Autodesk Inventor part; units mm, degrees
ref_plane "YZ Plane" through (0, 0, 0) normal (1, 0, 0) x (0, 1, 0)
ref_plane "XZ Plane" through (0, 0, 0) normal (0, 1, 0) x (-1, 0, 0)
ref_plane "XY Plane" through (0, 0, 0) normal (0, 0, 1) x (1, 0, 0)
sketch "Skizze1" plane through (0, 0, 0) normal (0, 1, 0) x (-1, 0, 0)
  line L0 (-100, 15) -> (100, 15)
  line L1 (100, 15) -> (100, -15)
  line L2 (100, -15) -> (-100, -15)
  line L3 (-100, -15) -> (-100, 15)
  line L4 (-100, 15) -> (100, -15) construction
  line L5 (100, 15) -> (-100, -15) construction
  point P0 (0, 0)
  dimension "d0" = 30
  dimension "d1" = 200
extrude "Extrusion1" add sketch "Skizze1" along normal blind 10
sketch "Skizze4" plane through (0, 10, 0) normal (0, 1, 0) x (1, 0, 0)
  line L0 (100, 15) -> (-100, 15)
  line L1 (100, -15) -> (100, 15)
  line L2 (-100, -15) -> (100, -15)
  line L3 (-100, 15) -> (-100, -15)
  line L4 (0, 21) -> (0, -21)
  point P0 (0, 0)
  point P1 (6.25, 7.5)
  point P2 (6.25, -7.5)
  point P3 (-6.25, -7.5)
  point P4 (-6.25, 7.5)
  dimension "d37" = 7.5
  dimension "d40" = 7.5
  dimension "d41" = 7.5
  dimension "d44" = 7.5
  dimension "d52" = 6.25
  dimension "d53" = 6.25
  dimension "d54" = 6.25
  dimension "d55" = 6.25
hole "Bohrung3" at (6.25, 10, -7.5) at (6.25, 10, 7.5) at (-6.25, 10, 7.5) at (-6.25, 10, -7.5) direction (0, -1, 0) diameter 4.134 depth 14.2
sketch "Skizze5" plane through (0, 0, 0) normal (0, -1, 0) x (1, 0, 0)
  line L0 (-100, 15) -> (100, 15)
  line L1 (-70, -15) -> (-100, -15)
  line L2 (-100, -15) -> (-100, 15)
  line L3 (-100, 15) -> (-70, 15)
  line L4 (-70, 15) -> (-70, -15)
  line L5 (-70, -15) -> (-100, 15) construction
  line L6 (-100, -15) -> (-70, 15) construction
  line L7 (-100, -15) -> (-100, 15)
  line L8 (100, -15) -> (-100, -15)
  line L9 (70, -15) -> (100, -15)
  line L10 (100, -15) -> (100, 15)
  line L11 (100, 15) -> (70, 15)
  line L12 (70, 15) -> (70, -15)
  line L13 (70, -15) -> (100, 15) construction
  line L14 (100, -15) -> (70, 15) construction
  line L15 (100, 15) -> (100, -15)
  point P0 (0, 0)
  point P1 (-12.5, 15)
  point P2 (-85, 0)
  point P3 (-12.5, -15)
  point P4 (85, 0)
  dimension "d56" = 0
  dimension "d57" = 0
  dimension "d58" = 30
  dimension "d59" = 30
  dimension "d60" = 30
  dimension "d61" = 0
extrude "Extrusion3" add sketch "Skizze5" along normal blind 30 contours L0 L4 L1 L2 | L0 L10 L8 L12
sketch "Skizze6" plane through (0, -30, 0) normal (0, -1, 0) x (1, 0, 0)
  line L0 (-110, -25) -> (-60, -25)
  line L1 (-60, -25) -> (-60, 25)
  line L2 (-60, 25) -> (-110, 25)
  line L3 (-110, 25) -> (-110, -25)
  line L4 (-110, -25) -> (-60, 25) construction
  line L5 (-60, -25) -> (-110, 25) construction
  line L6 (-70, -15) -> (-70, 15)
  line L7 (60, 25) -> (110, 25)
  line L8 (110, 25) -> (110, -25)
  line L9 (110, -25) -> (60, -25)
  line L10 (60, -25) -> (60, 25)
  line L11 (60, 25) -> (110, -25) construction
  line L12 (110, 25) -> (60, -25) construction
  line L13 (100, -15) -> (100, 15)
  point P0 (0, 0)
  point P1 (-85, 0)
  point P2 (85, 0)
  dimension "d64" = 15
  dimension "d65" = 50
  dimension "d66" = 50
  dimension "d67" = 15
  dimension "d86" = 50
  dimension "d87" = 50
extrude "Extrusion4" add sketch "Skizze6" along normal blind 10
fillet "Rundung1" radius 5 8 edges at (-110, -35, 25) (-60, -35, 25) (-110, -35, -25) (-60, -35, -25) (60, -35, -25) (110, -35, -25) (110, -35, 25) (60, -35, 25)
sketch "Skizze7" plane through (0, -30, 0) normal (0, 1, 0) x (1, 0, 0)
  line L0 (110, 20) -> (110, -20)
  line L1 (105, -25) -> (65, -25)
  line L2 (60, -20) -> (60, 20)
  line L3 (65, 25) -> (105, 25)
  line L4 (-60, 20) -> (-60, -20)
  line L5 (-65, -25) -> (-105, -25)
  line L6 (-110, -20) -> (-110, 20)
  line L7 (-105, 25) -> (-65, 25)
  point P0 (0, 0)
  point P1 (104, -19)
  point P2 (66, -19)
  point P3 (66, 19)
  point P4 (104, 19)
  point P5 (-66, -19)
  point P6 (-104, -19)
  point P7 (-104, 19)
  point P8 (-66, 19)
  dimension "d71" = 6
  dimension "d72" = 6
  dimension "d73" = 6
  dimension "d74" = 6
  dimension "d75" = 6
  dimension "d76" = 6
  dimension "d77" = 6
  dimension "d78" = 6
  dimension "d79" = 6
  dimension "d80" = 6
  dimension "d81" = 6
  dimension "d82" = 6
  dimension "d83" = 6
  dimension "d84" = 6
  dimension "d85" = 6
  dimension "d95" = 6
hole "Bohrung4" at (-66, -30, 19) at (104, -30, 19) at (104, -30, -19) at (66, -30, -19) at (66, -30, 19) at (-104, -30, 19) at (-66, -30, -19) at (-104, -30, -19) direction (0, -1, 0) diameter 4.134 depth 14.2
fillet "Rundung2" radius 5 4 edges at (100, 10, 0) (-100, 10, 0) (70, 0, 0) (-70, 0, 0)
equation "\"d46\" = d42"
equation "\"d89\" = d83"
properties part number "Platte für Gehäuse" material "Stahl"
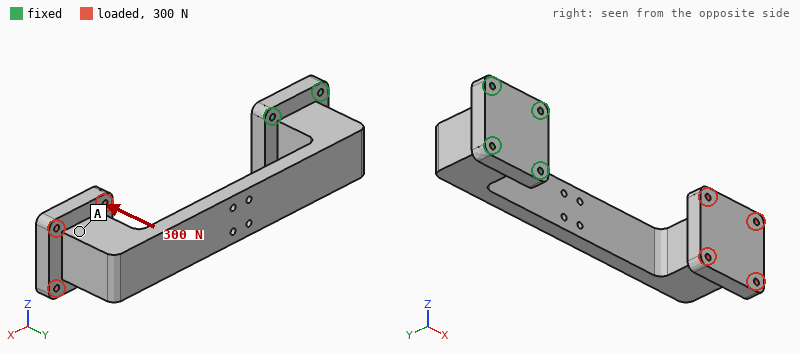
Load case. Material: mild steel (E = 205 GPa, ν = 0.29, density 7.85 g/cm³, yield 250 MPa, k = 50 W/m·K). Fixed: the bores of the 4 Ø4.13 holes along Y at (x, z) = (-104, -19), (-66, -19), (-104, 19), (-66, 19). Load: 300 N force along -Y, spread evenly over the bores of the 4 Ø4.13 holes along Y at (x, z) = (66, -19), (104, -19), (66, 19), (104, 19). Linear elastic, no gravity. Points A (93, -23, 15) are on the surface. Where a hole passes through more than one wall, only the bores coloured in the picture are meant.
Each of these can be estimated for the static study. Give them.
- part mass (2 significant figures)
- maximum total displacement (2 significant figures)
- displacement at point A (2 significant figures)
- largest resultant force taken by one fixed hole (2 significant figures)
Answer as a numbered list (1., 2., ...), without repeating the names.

1. 1.3 kg
2. 1.1 mm
3. 0.90 mm
4. 800 N
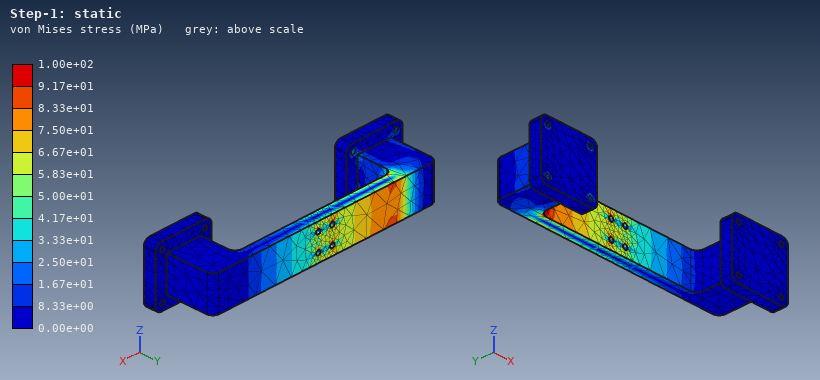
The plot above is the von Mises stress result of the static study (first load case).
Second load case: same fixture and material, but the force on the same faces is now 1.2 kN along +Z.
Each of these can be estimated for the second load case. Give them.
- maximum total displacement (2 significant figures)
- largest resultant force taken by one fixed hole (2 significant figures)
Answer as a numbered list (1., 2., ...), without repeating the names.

1. 1.2 mm
2. 2.1 kN
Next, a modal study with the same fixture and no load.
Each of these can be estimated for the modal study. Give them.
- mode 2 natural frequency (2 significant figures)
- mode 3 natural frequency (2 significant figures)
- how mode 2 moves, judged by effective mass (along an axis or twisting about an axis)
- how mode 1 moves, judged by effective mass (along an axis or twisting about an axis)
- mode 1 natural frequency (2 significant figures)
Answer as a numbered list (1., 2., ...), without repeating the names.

1. 280 Hz
2. 790 Hz
3. along Z
4. along Y
5. 130 Hz
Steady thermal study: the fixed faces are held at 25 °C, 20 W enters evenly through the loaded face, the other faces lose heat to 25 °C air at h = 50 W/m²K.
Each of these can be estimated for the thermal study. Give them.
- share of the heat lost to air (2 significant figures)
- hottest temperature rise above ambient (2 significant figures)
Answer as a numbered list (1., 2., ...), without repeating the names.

1. 97 %
2. 35 K
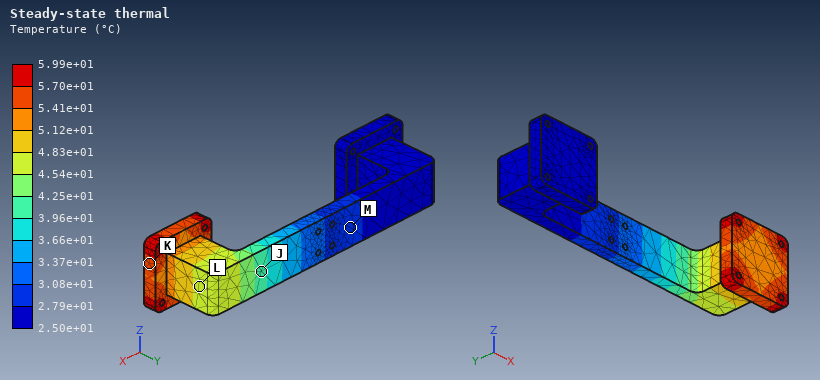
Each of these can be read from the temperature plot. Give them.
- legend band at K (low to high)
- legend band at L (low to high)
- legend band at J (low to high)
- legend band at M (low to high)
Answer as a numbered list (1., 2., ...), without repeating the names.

1. 5.41e+01 to 5.70e+01 °C
2. 4.54e+01 to 4.83e+01 °C
3. 3.96e+01 to 4.25e+01 °C
4. 2.79e+01 to 3.08e+01 °C
